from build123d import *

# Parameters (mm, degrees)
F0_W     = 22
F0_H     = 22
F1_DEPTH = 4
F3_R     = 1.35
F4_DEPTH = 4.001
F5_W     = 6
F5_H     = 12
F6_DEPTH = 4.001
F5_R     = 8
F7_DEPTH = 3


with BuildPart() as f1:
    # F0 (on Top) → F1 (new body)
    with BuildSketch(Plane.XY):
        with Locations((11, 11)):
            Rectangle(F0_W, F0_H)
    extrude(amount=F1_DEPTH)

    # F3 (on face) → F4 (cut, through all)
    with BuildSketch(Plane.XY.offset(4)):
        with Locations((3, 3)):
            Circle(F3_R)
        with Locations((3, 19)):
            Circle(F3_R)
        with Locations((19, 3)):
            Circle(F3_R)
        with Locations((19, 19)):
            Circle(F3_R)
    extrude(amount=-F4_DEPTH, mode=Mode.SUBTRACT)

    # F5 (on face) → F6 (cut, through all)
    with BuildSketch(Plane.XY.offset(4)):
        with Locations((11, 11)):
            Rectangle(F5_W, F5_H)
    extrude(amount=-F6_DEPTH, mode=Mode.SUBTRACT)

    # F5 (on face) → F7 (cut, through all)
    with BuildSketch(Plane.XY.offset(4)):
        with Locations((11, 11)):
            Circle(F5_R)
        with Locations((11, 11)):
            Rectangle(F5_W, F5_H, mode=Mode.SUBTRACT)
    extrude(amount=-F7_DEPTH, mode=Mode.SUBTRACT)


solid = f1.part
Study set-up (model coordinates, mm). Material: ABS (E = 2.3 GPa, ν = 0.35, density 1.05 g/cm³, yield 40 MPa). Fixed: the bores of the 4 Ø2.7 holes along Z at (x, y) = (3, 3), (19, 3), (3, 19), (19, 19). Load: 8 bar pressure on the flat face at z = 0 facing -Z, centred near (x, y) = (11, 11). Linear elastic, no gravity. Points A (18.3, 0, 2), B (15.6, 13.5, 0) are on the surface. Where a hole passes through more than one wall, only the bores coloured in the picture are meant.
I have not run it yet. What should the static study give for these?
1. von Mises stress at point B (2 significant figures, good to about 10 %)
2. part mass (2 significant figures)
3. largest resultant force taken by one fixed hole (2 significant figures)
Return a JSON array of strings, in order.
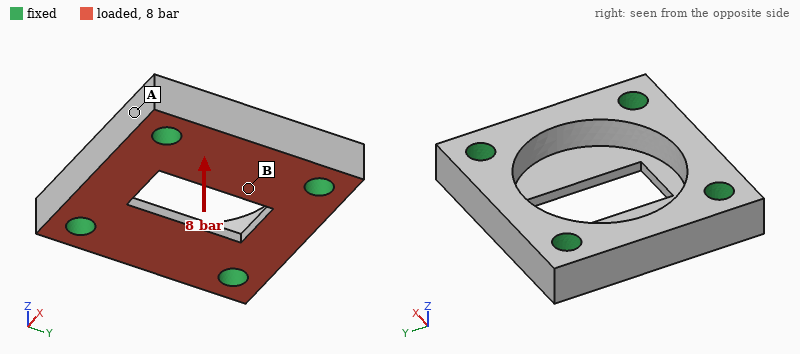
["11 MPa", "1.2 g", "78 N"]
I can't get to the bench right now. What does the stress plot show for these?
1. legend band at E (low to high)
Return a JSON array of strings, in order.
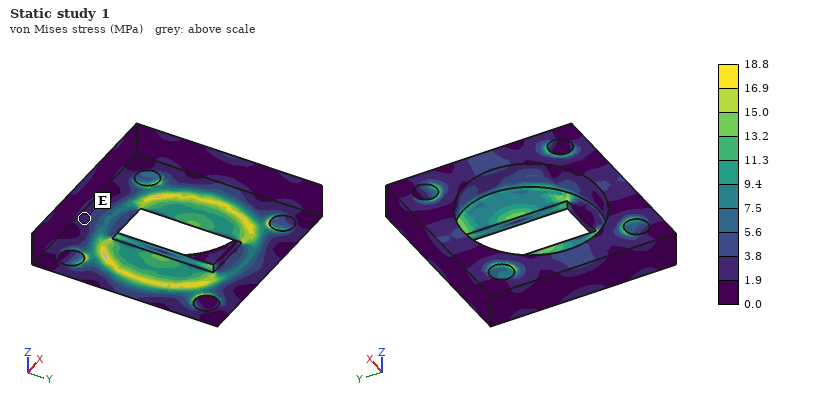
["1.9 to 3.8 MPa"]
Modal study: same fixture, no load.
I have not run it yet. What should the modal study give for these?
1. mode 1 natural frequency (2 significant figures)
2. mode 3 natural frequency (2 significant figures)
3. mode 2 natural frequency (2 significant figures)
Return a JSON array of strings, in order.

["13 kHz", "21 kHz", "13 kHz"]
